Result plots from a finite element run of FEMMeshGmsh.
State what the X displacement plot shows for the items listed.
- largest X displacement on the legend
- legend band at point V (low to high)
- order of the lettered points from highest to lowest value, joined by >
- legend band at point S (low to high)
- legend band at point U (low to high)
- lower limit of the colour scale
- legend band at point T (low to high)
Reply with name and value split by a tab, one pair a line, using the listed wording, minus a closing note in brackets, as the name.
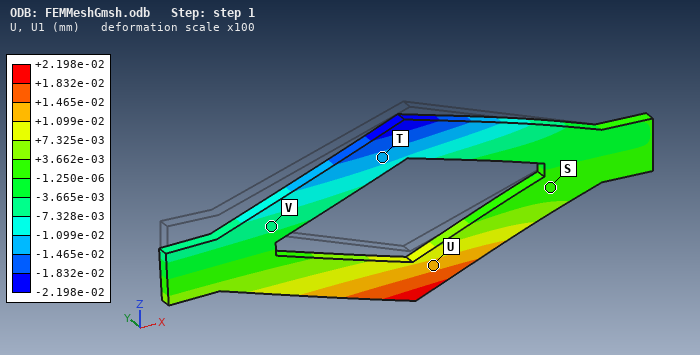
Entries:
largest X displacement on the legend	+2.198e-02 mm
legend band at point V	-7.328e-03 to -3.665e-03 mm
order of the lettered points from highest to lowest value, joined by >	U > S > V > T
legend band at point S	-1.250e-06 to +3.662e-03 mm
legend band at point U	+1.099e-02 to +1.465e-02 mm
lower limit of the colour scale	-2.198e-02 mm
legend band at point T	-1.465e-02 to -1.099e-02 mm
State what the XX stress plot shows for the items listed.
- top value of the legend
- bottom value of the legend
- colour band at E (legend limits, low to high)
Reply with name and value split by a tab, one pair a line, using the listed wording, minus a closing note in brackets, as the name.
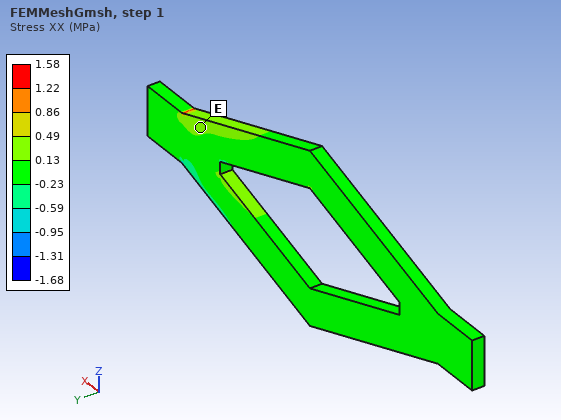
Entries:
top value of the legend	1.58 MPa
bottom value of the legend	-1.68 MPa
colour band at E	0.13 to 0.49 MPa
